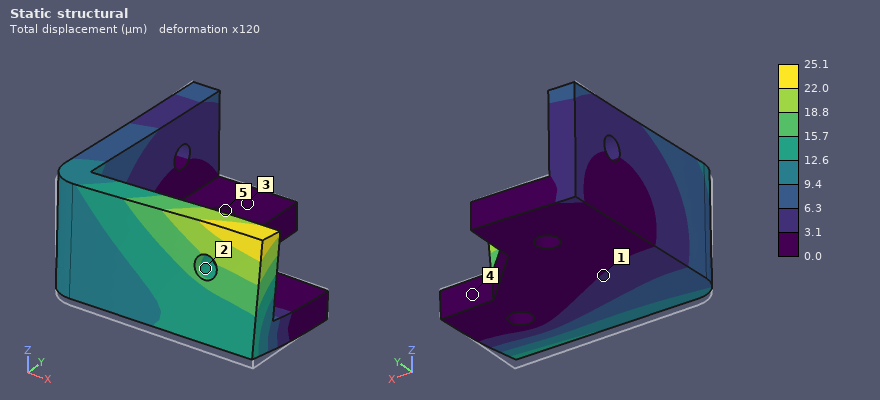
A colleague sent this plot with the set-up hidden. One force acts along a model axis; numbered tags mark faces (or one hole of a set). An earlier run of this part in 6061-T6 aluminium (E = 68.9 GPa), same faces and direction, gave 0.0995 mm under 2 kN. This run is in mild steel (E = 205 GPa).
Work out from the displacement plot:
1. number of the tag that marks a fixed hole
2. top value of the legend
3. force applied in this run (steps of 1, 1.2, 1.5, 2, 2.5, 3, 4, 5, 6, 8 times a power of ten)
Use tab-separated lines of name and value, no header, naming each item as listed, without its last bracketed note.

number of the tag that marks a fixed hole	5
top value of the legend	25.1 µm
force applied in this run	1.5 kN
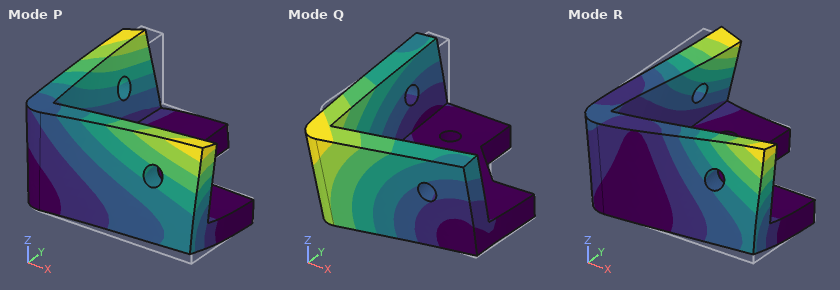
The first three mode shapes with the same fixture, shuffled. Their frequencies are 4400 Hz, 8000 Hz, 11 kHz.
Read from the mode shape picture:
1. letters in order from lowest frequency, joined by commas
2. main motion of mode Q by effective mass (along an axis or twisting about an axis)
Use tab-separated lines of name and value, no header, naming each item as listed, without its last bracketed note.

letters in order from lowest frequency, joined by commas	Q, P, R
main motion of mode Q by effective mass	along Z
